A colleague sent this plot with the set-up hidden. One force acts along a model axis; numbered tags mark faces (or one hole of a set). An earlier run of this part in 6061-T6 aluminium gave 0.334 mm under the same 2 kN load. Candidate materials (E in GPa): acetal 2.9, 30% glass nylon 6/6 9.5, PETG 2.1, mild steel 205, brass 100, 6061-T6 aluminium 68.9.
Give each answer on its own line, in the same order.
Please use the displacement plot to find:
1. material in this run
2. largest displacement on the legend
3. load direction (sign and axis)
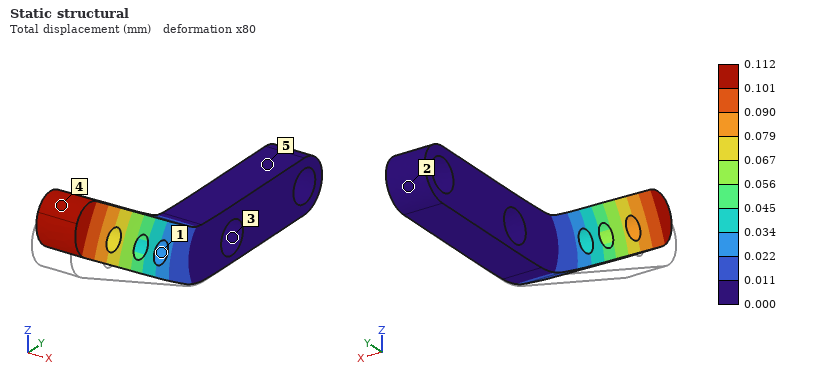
mild steel
0.112 mm
+Z
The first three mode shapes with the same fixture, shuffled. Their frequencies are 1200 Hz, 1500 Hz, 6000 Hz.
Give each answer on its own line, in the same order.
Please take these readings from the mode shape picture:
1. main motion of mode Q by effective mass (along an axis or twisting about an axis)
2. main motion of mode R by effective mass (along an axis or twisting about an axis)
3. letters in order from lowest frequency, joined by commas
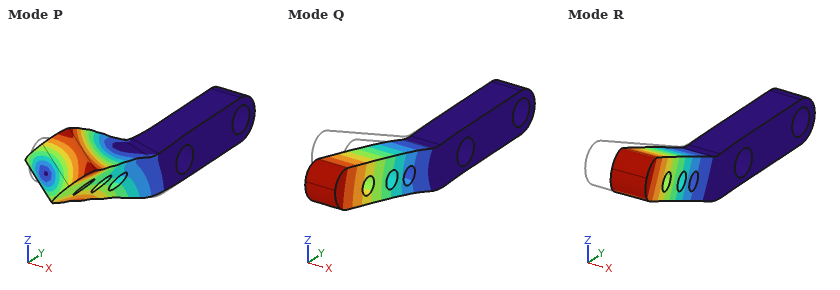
along Z
along X
R, Q, P
